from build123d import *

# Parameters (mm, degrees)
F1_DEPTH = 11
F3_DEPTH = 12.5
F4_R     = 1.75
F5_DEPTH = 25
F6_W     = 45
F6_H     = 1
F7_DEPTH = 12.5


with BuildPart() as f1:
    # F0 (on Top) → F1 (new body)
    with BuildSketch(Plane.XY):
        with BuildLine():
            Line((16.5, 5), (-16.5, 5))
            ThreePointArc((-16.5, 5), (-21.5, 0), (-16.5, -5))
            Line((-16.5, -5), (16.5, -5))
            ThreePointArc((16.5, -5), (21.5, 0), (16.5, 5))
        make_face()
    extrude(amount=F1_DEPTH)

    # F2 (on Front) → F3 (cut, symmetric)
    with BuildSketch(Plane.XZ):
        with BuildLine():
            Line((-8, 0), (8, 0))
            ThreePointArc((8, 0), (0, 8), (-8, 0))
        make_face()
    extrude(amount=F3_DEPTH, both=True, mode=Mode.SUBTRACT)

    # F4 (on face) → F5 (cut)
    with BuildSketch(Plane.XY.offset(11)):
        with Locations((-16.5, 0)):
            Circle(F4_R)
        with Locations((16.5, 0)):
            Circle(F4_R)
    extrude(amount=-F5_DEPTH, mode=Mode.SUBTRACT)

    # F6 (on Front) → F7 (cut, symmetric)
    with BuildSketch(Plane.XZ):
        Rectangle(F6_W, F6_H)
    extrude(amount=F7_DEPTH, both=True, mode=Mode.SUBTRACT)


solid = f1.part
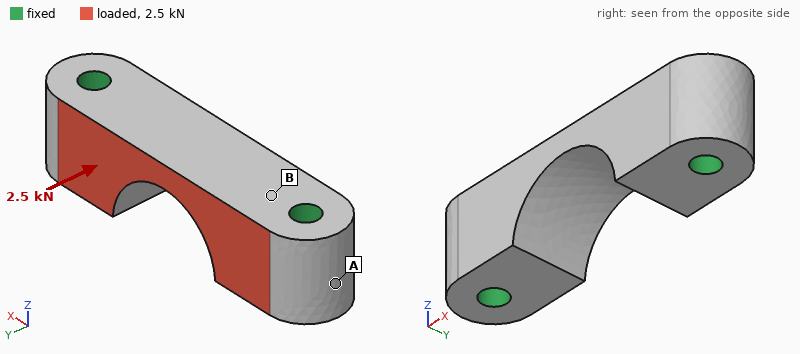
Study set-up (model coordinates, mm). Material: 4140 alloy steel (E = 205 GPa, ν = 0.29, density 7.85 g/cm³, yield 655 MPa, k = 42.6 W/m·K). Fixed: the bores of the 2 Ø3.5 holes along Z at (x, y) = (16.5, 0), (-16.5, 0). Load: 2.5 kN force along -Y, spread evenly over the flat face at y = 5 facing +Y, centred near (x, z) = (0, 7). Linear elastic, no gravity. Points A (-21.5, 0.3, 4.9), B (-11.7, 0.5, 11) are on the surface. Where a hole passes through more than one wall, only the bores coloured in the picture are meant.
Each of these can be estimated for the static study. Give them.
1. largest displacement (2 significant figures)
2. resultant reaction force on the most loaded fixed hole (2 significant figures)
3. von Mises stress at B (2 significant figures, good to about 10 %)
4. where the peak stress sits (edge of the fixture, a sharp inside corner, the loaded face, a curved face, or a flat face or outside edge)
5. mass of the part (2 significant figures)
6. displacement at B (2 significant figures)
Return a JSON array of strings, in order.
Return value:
["4.6 µm", "1.3 kN", "29 MPa", "edge of the fixture", "25 g", "1.4 µm"]
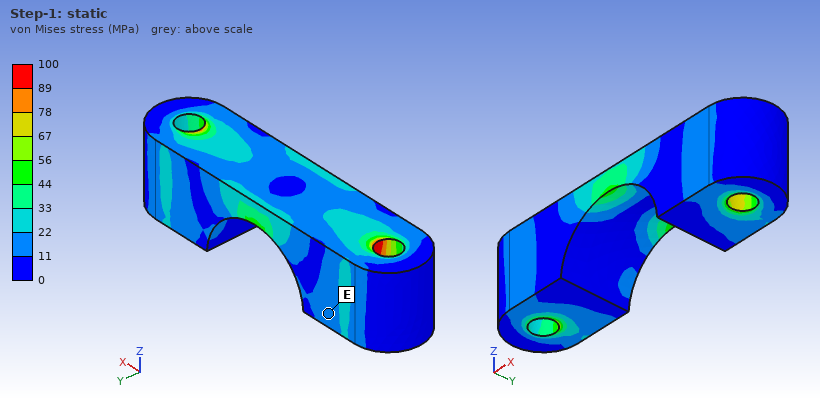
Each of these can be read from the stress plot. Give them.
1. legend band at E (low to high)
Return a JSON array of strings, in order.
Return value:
["11 to 22 MPa"]
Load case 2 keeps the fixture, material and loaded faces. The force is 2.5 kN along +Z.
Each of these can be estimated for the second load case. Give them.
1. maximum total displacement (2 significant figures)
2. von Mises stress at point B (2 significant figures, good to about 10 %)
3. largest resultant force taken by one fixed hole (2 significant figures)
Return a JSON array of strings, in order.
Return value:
["6.1 µm", "33 MPa", "1.3 kN"]
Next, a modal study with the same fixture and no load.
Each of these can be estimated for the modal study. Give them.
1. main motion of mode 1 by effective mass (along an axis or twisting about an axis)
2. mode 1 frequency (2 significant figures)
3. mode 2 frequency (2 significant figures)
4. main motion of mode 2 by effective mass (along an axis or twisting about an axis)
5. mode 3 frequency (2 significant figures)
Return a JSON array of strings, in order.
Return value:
["along Y", "33 kHz", "43 kHz", "along Z", "59 kHz"]
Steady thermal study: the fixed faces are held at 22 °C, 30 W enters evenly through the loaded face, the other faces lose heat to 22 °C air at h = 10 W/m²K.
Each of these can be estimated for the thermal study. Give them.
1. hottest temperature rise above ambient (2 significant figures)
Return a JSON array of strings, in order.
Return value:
["35 K"]
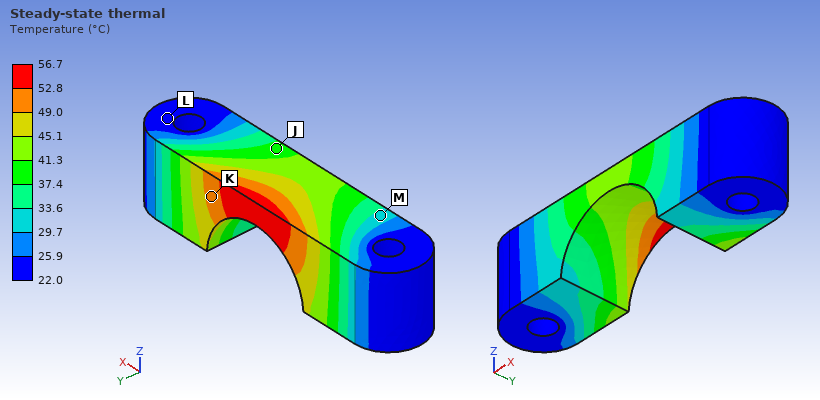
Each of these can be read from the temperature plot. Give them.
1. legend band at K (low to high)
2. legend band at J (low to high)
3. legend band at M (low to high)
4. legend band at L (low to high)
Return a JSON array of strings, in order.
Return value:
["49.0 to 52.8 °C", "37.4 to 41.3 °C", "29.7 to 33.6 °C", "22.0 to 25.9 °C"]
